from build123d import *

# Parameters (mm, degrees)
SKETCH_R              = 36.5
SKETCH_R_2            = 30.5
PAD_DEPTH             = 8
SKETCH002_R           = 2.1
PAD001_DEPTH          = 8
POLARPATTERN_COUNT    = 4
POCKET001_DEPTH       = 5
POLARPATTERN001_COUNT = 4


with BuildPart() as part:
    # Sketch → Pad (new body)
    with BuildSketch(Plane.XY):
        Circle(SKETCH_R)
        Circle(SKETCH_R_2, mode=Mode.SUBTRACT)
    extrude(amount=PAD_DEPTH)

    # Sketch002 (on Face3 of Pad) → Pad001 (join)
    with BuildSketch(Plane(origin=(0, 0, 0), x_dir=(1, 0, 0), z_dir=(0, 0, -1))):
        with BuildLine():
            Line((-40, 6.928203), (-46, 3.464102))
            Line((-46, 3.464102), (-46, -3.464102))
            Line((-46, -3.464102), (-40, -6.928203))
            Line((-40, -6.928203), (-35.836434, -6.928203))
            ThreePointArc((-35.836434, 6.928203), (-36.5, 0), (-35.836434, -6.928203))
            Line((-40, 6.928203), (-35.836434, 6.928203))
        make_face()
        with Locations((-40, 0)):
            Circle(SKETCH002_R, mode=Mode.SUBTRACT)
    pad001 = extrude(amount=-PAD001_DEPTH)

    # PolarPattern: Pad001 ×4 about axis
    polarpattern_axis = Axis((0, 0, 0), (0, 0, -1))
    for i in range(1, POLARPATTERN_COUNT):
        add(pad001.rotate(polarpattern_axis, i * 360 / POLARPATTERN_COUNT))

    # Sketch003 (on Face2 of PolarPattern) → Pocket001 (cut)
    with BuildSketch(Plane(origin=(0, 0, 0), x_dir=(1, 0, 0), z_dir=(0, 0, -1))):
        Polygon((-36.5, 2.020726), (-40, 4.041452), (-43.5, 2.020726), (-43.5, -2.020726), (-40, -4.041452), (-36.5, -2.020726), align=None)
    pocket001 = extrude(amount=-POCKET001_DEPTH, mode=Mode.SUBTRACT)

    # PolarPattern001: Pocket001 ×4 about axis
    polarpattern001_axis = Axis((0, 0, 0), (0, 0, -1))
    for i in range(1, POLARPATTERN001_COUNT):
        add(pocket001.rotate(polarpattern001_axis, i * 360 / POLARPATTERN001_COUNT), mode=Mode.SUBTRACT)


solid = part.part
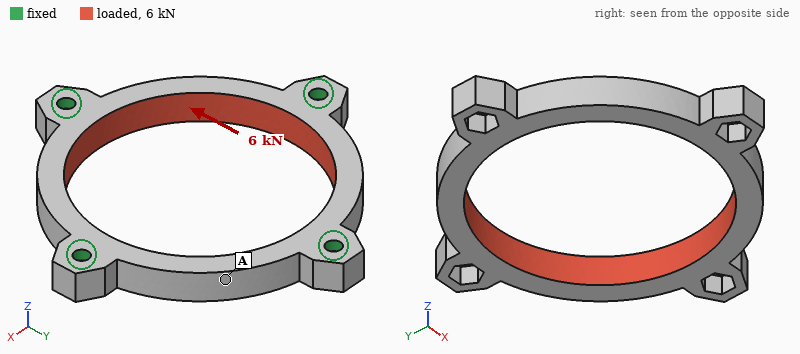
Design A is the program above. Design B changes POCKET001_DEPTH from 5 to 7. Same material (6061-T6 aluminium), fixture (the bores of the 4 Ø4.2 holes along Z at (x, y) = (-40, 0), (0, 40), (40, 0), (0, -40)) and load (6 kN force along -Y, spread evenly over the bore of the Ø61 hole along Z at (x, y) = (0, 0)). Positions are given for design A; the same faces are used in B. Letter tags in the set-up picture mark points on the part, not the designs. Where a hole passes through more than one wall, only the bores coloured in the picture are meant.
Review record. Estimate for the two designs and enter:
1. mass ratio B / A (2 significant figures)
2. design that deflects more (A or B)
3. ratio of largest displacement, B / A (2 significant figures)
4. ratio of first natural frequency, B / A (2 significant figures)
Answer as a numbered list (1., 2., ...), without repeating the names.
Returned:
1. 0.98
2. B
3. 1.8
4. 0.68
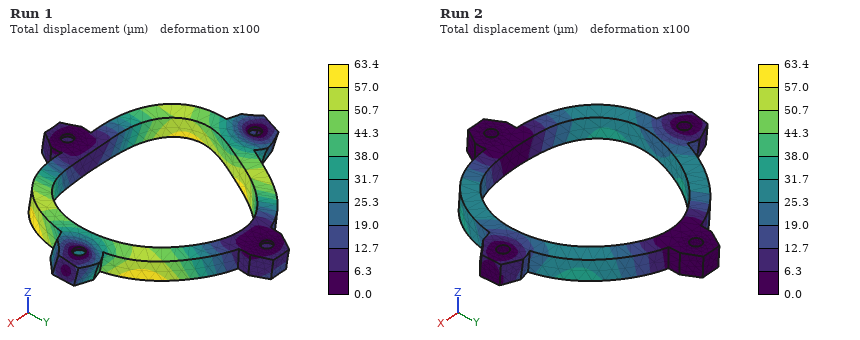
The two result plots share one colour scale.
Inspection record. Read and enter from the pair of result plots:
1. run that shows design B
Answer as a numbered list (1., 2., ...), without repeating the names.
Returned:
1. Run 1
